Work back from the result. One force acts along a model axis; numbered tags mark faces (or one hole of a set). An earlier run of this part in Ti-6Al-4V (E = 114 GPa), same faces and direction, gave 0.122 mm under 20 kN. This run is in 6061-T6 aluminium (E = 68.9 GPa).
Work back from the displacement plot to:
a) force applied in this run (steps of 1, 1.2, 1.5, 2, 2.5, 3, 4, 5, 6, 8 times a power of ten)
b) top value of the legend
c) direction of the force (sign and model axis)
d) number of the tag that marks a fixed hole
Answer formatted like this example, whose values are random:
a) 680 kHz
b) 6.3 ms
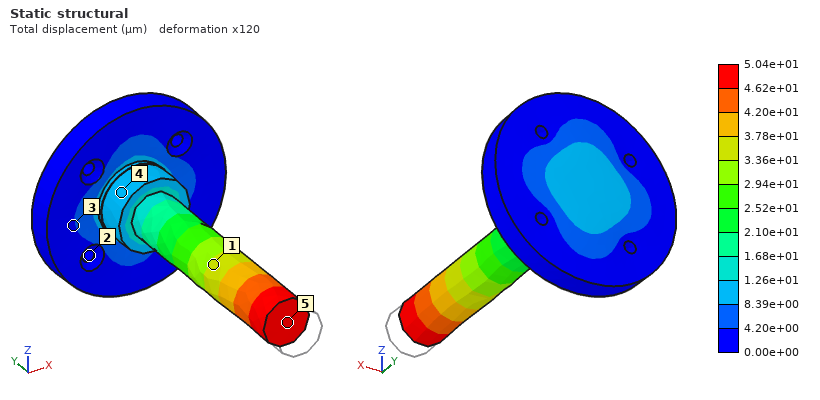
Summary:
a) 5 kN
b) 5.04e+01 µm
c) +Y
d) 2
